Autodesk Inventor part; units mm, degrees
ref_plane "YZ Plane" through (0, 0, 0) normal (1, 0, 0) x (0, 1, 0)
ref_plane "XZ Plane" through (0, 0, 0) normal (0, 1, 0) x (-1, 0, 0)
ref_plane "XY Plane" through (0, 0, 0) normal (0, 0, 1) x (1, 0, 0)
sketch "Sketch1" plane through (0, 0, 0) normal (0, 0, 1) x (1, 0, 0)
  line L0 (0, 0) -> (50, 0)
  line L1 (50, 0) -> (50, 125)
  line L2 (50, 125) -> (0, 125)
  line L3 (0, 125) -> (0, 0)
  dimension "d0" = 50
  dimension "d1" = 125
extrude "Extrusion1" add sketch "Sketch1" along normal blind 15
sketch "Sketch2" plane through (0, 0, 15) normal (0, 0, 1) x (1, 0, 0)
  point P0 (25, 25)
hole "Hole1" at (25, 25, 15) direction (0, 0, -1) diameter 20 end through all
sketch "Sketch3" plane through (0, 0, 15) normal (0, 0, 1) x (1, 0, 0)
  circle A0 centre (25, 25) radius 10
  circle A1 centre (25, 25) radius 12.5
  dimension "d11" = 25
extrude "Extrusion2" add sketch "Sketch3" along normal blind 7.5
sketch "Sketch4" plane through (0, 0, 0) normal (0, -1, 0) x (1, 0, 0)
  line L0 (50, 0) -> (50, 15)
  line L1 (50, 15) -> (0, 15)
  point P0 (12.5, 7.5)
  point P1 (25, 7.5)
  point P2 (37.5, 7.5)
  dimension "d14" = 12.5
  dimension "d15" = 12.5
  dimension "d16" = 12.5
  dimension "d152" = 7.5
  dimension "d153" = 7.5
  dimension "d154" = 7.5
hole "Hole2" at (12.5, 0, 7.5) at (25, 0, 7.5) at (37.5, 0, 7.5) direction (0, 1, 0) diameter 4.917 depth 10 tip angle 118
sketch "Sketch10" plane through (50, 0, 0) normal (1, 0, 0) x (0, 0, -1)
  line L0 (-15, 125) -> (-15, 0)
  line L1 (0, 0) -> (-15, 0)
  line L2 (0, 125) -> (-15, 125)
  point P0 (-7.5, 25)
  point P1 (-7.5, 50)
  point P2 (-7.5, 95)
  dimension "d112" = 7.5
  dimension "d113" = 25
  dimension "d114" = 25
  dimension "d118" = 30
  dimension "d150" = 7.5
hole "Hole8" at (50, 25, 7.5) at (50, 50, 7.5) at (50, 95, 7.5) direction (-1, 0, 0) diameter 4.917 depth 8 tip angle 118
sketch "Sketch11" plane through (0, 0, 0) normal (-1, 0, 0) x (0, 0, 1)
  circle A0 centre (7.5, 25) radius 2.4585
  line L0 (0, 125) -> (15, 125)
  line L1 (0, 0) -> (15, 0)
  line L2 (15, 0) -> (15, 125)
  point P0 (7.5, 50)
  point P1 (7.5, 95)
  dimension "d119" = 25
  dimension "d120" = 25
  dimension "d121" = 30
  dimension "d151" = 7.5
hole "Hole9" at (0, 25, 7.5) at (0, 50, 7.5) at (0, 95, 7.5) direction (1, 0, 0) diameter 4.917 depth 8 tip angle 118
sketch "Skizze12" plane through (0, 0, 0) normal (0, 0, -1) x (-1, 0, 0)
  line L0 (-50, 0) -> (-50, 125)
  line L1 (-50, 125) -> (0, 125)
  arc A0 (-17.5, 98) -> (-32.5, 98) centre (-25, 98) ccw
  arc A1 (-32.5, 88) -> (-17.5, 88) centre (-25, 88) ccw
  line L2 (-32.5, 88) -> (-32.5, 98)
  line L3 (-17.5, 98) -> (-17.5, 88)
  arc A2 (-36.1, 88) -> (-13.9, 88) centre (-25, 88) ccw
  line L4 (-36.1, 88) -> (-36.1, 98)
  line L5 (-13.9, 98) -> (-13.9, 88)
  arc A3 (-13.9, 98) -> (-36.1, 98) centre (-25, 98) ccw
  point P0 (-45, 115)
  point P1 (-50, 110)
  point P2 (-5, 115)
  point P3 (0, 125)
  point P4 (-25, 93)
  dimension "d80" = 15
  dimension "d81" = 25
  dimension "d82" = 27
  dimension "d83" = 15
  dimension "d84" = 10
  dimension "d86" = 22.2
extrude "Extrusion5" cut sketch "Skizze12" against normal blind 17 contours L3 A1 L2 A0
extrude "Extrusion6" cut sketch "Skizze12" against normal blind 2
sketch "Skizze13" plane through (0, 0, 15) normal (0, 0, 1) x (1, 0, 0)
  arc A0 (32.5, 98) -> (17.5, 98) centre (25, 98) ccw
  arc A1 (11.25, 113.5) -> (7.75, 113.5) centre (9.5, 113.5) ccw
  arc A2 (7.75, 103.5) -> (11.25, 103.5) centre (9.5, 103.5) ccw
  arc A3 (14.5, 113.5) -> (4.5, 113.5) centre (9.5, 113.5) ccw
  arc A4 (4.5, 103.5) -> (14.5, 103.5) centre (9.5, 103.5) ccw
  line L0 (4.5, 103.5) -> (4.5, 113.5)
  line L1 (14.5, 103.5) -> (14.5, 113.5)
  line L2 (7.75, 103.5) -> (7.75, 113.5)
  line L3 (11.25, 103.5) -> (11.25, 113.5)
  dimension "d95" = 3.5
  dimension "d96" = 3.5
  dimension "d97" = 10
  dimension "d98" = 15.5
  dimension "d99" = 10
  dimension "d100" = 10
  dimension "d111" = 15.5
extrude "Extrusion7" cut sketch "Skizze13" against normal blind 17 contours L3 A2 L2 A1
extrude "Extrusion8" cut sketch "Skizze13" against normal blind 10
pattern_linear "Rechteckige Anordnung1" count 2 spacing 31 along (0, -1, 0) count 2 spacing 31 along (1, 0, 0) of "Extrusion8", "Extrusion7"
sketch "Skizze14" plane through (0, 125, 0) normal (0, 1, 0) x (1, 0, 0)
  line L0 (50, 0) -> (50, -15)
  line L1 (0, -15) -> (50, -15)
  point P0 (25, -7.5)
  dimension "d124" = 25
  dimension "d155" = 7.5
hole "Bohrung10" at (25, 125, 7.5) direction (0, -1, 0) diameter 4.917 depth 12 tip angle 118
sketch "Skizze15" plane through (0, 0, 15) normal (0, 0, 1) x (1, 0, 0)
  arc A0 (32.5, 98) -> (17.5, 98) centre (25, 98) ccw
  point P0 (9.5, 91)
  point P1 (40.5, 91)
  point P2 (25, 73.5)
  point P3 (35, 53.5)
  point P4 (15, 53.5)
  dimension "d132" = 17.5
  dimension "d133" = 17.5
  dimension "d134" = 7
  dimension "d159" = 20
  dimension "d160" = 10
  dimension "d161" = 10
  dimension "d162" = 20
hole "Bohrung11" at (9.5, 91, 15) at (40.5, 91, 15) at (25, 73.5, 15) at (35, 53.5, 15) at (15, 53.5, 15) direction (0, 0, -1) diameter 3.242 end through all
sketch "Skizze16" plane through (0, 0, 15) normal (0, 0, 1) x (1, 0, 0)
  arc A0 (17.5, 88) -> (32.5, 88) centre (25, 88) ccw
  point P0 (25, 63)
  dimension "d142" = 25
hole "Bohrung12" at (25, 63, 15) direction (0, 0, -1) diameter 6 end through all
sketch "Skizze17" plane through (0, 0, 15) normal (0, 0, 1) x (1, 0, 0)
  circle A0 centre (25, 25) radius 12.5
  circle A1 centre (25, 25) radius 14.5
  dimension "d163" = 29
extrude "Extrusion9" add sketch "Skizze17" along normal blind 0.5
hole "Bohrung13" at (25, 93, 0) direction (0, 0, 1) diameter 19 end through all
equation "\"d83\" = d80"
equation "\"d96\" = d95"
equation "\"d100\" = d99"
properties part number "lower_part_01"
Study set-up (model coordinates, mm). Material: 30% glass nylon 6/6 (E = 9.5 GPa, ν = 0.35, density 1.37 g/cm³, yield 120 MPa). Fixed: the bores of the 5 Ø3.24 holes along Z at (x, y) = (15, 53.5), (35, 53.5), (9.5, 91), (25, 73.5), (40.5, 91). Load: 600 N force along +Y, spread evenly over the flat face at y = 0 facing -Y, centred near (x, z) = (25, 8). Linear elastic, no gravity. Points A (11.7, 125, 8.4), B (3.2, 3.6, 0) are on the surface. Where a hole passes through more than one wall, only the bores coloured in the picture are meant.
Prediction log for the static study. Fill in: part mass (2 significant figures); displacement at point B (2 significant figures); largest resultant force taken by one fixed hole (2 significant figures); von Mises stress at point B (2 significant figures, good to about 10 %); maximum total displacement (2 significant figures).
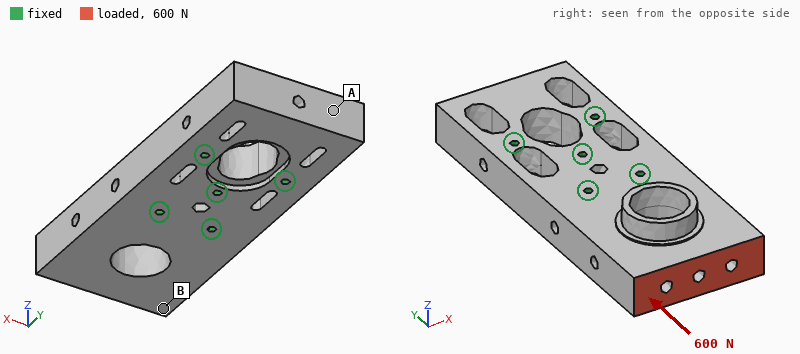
100 g
6.7 µm
240 N
0.88 MPa
9.7 µm
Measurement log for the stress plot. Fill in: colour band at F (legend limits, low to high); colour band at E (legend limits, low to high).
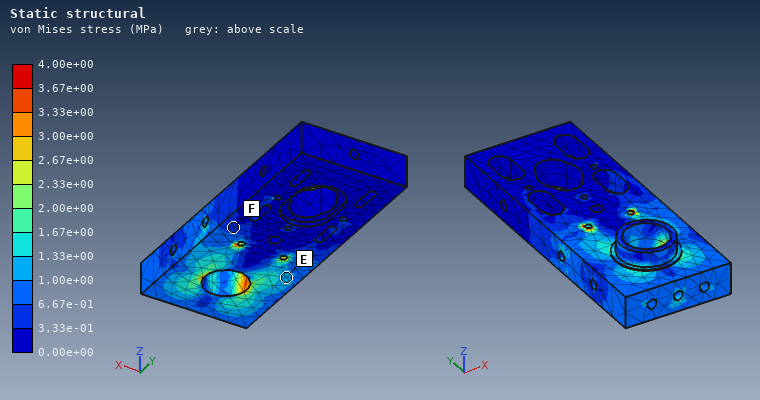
3.33e-01 to 6.67e-01 MPa
1.00e+00 to 1.33e+00 MPa
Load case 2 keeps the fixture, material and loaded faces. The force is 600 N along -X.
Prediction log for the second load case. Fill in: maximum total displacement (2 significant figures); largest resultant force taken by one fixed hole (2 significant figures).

81 µm
960 N
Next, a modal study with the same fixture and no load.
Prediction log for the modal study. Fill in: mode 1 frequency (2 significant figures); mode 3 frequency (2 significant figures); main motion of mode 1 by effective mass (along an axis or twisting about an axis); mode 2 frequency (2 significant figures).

1900 Hz
3500 Hz
along Z
3400 Hz
